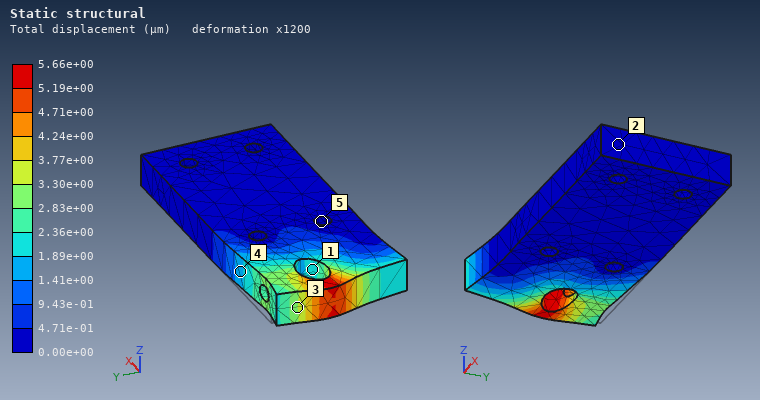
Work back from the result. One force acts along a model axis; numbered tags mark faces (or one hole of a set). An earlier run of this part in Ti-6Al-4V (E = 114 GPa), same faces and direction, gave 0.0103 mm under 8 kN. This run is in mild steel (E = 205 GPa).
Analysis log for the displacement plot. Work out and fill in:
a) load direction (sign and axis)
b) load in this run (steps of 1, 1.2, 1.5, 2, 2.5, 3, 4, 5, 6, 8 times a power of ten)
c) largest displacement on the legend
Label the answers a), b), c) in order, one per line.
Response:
a) -X
b) 8 kN
c) 5.66e+00 µm
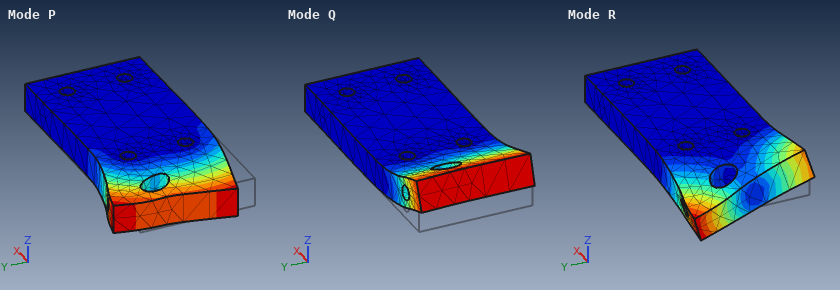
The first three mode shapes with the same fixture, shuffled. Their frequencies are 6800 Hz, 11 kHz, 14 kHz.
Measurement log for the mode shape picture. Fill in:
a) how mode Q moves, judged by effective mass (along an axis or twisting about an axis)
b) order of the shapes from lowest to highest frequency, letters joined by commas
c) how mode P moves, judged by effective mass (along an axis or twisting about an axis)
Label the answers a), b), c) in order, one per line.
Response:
a) along Z
b) Q, R, P
c) along Y
